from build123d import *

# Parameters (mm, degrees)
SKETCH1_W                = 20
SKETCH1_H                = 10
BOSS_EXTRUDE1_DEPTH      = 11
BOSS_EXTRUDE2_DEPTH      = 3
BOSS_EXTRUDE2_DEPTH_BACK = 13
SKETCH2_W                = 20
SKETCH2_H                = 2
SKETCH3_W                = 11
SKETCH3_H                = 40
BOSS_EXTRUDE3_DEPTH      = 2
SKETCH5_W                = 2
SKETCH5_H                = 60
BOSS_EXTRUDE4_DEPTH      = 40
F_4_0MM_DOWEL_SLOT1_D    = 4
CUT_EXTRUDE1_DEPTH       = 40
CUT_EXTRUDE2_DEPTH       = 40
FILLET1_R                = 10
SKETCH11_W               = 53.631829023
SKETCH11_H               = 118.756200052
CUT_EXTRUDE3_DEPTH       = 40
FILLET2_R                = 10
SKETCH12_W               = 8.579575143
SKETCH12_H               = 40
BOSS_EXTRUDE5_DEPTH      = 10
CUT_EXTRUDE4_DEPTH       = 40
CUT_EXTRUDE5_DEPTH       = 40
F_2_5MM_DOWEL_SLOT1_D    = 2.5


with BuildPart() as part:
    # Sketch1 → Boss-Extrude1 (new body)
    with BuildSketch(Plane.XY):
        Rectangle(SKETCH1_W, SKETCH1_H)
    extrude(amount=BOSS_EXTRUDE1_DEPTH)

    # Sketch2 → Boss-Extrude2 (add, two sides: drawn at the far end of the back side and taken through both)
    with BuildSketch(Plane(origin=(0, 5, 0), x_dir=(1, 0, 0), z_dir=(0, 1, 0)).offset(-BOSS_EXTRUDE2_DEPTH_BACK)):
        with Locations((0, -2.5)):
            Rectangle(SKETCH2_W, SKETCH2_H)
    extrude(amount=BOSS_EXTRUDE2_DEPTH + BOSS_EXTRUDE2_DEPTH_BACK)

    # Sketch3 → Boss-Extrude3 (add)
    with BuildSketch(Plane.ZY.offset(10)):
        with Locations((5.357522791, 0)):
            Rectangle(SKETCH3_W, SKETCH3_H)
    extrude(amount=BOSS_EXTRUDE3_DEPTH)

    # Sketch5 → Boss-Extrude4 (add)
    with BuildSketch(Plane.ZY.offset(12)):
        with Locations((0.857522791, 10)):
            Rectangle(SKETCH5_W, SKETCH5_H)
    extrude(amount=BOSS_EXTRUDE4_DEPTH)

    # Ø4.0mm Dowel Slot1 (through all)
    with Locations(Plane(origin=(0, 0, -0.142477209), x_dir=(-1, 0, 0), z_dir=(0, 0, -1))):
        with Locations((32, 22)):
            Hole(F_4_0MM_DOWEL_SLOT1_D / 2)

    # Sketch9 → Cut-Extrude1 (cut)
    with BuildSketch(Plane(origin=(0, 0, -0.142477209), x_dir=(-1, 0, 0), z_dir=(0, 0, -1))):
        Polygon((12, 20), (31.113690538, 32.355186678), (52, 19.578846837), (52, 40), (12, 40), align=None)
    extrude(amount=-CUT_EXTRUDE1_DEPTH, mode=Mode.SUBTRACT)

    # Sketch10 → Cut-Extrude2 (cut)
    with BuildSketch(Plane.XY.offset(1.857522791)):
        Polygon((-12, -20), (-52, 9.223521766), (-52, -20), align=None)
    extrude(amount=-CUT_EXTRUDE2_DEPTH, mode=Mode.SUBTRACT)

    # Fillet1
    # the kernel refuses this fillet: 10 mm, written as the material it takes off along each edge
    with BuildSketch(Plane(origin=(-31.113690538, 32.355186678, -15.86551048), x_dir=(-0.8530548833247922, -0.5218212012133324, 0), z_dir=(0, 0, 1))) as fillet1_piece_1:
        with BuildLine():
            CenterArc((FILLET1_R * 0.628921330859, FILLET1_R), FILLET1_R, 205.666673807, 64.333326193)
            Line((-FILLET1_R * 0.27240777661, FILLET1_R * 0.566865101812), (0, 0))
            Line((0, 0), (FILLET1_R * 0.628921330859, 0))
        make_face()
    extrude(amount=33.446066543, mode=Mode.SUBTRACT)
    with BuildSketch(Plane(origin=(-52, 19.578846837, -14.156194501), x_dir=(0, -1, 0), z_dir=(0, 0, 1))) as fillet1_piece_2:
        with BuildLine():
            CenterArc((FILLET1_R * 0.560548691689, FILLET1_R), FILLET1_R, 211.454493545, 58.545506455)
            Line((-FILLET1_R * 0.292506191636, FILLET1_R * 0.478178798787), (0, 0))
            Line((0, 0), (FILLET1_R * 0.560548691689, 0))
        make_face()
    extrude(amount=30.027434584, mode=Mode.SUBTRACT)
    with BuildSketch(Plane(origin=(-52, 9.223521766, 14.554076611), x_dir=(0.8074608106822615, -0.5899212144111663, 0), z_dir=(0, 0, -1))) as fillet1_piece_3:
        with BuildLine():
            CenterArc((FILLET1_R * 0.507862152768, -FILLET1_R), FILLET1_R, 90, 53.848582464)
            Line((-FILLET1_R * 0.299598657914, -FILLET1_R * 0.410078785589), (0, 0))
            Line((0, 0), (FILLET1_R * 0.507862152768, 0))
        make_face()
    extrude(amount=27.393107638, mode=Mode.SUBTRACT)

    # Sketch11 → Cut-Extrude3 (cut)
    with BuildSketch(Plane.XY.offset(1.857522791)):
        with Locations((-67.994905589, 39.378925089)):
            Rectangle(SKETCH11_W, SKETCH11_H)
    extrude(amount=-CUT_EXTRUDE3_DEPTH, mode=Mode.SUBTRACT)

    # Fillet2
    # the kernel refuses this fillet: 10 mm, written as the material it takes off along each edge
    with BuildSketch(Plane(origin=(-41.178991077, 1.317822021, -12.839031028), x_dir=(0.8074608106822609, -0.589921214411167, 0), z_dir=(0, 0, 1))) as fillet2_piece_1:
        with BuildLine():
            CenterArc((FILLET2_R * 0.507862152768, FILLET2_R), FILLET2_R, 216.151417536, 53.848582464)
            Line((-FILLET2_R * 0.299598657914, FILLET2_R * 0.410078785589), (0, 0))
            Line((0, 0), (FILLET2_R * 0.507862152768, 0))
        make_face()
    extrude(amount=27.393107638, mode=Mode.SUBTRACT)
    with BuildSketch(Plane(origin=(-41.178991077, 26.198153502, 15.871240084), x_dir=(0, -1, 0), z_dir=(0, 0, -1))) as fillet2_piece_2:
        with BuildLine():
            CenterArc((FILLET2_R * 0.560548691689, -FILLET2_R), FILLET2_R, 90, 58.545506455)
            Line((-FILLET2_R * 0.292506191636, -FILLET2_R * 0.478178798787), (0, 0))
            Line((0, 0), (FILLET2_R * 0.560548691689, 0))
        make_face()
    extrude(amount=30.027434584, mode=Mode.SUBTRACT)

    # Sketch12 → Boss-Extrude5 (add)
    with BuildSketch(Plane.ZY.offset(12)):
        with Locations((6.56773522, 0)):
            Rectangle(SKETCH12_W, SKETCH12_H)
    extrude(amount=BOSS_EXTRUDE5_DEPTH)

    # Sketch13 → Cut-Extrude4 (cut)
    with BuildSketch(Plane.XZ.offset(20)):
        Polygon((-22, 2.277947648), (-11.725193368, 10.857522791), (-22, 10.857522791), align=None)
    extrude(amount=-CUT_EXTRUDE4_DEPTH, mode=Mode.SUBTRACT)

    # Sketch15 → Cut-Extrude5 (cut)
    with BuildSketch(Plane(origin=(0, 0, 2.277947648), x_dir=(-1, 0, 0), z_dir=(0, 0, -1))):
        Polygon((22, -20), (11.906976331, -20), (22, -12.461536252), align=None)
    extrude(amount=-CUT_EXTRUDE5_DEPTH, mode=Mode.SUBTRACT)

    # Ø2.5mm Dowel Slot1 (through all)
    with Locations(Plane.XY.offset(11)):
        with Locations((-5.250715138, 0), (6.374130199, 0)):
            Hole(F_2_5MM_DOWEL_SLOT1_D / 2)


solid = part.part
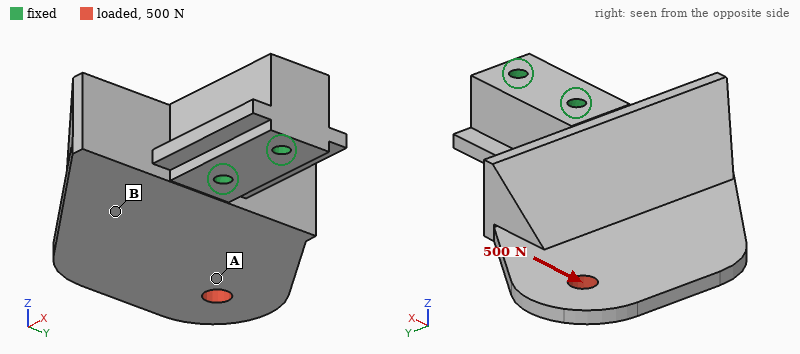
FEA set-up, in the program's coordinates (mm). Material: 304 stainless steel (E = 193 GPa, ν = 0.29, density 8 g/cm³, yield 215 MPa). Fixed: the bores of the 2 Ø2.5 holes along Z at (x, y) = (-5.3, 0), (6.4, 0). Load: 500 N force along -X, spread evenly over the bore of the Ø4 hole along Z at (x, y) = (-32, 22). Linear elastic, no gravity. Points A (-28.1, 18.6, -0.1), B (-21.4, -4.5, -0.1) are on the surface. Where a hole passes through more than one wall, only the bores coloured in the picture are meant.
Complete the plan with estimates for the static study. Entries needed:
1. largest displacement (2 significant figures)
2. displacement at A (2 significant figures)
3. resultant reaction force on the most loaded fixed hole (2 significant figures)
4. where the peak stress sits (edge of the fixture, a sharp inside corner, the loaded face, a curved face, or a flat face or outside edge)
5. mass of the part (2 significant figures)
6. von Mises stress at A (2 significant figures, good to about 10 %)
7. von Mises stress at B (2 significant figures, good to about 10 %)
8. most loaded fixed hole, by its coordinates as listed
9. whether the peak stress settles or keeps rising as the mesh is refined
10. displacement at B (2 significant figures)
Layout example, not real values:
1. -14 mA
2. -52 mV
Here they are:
1. 40 µm
2. 25 µm
3. 780 N
4. a sharp inside corner
5. 55 g
6. 23 MPa
7. 9.4 MPa
8. (-5.3, 0)
9. keeps rising
10. 9.3 µm
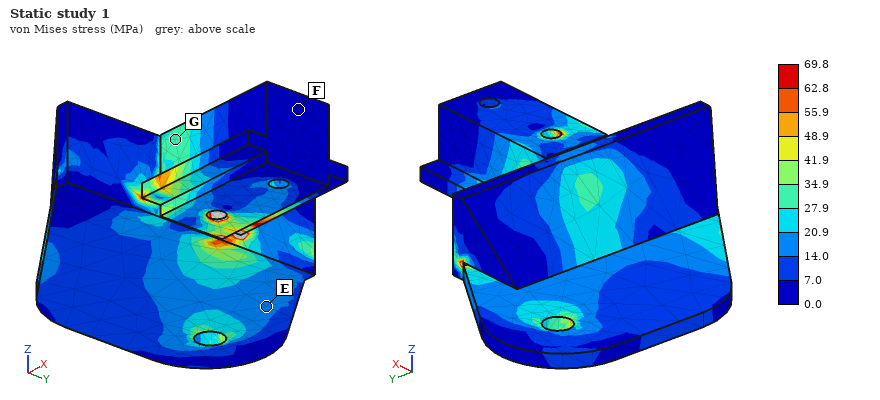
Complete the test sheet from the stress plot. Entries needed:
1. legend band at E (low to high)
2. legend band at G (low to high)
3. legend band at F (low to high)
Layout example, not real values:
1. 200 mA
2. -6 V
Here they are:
1. 14.0 to 20.9 MPa
2. 27.9 to 34.9 MPa
3. 0.0 to 7.0 MPa
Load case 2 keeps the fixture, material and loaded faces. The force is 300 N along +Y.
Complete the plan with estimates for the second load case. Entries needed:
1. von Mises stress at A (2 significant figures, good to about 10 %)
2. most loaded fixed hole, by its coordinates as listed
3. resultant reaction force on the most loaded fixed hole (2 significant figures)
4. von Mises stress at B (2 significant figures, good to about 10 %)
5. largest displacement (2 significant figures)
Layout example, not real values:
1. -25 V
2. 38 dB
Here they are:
1. 11 MPa
2. (-5.3, 0)
3. 770 N
4. 9.1 MPa
5. 23 µm
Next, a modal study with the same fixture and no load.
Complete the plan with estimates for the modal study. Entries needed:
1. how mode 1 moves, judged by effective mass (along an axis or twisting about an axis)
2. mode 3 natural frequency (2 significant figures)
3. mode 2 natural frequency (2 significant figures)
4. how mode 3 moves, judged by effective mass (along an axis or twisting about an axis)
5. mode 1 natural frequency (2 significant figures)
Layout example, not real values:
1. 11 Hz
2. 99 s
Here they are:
1. along Z
2. 5500 Hz
3. 4000 Hz
4. along Y
5. 1600 Hz
